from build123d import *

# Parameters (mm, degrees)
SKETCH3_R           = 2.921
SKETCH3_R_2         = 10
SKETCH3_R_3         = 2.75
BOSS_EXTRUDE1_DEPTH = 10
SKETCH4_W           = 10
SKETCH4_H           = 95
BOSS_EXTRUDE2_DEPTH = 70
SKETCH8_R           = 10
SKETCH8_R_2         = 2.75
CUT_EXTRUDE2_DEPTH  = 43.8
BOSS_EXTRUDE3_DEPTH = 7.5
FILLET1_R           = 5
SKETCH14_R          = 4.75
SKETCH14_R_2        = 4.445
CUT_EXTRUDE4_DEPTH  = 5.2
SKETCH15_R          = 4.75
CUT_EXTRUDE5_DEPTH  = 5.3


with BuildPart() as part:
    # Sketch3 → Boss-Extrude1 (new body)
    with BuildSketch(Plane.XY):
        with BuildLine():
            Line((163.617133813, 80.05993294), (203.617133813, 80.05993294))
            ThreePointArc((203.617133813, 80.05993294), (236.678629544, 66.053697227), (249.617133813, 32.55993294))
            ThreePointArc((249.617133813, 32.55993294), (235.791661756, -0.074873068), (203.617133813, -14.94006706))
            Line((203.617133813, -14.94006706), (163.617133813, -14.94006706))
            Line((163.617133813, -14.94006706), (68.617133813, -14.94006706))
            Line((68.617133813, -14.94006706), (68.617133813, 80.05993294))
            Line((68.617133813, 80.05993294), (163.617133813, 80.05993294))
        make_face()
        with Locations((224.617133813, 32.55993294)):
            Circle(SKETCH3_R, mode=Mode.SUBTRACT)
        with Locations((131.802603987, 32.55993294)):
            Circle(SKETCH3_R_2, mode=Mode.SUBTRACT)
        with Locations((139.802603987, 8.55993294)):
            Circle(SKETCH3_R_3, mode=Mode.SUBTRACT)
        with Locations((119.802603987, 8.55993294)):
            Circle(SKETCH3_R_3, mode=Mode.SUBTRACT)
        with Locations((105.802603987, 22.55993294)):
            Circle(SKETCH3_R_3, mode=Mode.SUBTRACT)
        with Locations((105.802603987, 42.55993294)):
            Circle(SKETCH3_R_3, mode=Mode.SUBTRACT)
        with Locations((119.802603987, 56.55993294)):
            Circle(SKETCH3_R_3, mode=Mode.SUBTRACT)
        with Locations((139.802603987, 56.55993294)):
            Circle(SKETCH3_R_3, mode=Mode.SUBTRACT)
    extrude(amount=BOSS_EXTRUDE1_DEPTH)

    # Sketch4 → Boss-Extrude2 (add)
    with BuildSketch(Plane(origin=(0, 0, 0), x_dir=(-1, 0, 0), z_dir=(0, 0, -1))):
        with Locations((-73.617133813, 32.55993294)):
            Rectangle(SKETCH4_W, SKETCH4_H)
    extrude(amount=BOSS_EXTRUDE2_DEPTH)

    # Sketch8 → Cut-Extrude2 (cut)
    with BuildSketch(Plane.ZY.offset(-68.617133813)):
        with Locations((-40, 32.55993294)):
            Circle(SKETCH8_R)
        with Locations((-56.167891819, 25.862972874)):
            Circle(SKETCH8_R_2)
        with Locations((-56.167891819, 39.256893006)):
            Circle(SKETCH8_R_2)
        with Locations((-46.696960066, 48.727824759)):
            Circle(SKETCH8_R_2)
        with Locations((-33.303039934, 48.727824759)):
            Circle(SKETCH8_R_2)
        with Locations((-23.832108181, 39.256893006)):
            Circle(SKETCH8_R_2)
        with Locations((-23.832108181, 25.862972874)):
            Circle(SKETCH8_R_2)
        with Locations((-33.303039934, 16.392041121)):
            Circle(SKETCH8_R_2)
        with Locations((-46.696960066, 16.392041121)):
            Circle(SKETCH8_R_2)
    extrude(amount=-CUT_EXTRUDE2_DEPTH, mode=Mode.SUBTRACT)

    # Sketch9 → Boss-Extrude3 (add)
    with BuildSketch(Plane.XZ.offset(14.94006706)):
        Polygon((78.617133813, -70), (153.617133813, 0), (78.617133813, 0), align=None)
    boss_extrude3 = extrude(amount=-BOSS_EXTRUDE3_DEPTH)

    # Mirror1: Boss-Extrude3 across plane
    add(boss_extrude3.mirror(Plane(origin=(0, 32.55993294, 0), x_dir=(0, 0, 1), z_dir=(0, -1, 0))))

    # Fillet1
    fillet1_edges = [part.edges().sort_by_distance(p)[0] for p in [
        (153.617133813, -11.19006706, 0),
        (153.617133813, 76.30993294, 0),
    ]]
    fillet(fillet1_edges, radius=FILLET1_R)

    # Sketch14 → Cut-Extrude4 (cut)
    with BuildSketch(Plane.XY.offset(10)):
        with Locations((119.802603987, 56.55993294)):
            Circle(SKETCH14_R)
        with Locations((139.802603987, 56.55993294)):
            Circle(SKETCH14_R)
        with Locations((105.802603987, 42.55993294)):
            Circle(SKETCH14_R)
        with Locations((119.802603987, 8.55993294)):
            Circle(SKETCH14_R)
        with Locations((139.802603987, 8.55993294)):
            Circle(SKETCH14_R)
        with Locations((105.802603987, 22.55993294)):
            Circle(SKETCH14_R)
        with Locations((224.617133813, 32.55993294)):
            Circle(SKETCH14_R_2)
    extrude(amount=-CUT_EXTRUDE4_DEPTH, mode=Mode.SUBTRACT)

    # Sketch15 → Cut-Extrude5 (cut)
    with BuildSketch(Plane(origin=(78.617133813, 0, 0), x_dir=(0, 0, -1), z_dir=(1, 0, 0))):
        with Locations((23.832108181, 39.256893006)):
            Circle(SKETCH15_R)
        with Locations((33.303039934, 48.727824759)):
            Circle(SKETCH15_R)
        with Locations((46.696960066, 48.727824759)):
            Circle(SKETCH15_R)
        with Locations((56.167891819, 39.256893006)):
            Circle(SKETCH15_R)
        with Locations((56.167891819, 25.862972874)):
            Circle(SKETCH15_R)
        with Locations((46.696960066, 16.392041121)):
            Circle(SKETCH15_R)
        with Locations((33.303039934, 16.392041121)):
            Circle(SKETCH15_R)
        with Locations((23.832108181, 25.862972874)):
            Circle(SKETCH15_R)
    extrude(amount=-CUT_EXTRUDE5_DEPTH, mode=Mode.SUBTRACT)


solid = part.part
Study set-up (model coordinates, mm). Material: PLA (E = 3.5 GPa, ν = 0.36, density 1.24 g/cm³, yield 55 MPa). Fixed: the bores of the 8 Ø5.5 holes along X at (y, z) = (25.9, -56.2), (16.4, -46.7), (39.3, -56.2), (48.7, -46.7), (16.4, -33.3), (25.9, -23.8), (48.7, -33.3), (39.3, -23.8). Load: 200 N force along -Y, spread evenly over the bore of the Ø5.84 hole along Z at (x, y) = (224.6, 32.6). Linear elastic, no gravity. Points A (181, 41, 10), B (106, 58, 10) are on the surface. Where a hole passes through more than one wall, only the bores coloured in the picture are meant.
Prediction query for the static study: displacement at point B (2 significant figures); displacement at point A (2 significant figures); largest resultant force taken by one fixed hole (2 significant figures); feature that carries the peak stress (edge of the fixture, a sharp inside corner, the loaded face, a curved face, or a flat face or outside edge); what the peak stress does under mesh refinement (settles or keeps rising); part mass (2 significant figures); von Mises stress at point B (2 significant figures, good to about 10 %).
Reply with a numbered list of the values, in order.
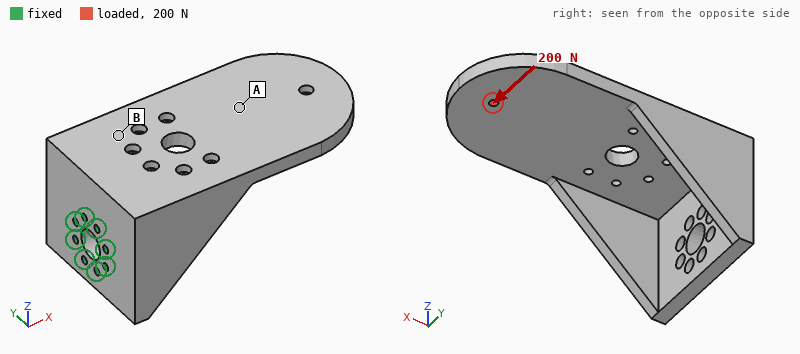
1. 0.56 mm
2. 1.4 mm
3. 520 N
4. edge of the fixture
5. keeps rising
6. 320 g
7. 3.3 MPa
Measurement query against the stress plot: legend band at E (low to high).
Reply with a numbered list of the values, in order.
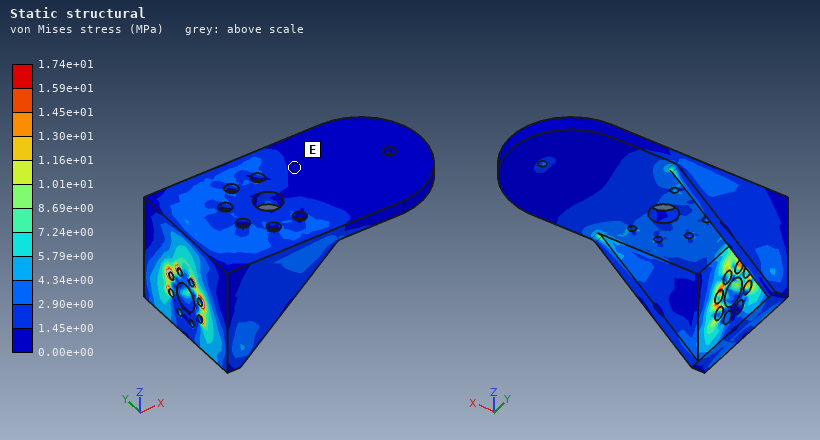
1. 0.00e+00 to 1.45e+00 MPa
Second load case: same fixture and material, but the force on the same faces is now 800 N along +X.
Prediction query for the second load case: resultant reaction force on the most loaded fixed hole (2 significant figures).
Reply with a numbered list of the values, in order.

1. 580 N
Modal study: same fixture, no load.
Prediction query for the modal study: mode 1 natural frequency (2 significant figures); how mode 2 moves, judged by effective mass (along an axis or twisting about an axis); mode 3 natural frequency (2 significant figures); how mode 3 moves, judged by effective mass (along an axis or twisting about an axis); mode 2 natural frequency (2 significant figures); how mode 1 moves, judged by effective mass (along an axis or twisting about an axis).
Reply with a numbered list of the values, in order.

1. 140 Hz
2. along Y
3. 470 Hz
4. along X
5. 170 Hz
6. along Z
